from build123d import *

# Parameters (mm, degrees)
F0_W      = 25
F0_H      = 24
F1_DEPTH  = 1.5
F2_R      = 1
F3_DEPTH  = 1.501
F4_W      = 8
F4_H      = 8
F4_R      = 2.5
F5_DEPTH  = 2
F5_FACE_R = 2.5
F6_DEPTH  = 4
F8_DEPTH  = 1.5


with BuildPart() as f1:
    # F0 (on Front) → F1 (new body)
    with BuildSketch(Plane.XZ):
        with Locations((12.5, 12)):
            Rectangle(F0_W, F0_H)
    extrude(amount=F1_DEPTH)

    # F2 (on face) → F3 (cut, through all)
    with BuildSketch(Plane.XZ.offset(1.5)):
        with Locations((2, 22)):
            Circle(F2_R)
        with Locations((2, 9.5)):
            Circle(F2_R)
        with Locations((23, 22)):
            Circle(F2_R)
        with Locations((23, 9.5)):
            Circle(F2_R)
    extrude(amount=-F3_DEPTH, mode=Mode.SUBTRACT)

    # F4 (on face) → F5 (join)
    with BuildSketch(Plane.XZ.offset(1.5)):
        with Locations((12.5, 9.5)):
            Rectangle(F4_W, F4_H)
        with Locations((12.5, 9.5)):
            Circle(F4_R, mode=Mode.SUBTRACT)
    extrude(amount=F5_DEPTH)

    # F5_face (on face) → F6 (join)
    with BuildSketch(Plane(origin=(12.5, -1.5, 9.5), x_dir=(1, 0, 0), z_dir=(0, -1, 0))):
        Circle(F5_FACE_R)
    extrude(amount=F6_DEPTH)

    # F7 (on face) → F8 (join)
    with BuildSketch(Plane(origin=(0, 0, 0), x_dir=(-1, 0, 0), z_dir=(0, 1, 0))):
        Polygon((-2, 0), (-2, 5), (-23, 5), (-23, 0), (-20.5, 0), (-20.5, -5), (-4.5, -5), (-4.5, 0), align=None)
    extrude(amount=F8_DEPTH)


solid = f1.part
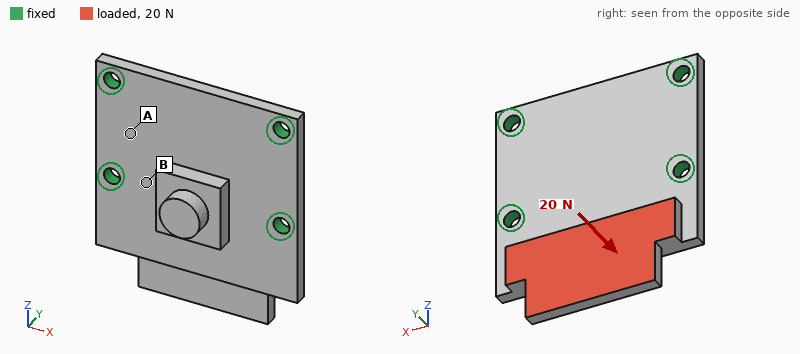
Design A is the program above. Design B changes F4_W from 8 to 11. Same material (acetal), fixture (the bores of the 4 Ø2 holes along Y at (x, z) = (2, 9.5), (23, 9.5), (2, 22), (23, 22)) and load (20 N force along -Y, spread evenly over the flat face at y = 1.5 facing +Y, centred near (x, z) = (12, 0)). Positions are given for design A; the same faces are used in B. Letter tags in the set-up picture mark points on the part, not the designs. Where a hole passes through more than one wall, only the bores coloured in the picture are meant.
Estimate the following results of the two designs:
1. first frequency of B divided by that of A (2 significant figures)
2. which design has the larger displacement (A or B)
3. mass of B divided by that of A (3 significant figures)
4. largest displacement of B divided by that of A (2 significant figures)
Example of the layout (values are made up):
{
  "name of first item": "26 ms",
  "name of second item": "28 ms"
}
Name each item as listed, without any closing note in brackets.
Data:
{
  "first frequency of B divided by that of A": "1.0",
  "which design has the larger displacement": "A",
  "mass of B divided by that of A": "1.04",
  "largest displacement of B divided by that of A": "0.91"
}
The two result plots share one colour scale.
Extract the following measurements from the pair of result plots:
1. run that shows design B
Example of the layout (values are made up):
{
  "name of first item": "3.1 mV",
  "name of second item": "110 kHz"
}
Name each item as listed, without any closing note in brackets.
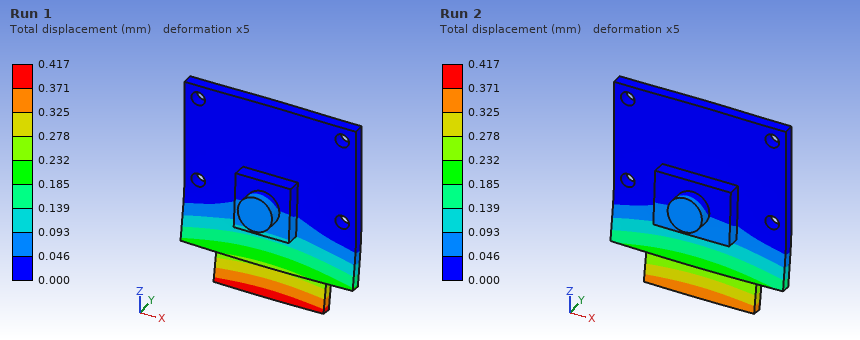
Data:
{
  "run that shows design B": "Run 2"
}
